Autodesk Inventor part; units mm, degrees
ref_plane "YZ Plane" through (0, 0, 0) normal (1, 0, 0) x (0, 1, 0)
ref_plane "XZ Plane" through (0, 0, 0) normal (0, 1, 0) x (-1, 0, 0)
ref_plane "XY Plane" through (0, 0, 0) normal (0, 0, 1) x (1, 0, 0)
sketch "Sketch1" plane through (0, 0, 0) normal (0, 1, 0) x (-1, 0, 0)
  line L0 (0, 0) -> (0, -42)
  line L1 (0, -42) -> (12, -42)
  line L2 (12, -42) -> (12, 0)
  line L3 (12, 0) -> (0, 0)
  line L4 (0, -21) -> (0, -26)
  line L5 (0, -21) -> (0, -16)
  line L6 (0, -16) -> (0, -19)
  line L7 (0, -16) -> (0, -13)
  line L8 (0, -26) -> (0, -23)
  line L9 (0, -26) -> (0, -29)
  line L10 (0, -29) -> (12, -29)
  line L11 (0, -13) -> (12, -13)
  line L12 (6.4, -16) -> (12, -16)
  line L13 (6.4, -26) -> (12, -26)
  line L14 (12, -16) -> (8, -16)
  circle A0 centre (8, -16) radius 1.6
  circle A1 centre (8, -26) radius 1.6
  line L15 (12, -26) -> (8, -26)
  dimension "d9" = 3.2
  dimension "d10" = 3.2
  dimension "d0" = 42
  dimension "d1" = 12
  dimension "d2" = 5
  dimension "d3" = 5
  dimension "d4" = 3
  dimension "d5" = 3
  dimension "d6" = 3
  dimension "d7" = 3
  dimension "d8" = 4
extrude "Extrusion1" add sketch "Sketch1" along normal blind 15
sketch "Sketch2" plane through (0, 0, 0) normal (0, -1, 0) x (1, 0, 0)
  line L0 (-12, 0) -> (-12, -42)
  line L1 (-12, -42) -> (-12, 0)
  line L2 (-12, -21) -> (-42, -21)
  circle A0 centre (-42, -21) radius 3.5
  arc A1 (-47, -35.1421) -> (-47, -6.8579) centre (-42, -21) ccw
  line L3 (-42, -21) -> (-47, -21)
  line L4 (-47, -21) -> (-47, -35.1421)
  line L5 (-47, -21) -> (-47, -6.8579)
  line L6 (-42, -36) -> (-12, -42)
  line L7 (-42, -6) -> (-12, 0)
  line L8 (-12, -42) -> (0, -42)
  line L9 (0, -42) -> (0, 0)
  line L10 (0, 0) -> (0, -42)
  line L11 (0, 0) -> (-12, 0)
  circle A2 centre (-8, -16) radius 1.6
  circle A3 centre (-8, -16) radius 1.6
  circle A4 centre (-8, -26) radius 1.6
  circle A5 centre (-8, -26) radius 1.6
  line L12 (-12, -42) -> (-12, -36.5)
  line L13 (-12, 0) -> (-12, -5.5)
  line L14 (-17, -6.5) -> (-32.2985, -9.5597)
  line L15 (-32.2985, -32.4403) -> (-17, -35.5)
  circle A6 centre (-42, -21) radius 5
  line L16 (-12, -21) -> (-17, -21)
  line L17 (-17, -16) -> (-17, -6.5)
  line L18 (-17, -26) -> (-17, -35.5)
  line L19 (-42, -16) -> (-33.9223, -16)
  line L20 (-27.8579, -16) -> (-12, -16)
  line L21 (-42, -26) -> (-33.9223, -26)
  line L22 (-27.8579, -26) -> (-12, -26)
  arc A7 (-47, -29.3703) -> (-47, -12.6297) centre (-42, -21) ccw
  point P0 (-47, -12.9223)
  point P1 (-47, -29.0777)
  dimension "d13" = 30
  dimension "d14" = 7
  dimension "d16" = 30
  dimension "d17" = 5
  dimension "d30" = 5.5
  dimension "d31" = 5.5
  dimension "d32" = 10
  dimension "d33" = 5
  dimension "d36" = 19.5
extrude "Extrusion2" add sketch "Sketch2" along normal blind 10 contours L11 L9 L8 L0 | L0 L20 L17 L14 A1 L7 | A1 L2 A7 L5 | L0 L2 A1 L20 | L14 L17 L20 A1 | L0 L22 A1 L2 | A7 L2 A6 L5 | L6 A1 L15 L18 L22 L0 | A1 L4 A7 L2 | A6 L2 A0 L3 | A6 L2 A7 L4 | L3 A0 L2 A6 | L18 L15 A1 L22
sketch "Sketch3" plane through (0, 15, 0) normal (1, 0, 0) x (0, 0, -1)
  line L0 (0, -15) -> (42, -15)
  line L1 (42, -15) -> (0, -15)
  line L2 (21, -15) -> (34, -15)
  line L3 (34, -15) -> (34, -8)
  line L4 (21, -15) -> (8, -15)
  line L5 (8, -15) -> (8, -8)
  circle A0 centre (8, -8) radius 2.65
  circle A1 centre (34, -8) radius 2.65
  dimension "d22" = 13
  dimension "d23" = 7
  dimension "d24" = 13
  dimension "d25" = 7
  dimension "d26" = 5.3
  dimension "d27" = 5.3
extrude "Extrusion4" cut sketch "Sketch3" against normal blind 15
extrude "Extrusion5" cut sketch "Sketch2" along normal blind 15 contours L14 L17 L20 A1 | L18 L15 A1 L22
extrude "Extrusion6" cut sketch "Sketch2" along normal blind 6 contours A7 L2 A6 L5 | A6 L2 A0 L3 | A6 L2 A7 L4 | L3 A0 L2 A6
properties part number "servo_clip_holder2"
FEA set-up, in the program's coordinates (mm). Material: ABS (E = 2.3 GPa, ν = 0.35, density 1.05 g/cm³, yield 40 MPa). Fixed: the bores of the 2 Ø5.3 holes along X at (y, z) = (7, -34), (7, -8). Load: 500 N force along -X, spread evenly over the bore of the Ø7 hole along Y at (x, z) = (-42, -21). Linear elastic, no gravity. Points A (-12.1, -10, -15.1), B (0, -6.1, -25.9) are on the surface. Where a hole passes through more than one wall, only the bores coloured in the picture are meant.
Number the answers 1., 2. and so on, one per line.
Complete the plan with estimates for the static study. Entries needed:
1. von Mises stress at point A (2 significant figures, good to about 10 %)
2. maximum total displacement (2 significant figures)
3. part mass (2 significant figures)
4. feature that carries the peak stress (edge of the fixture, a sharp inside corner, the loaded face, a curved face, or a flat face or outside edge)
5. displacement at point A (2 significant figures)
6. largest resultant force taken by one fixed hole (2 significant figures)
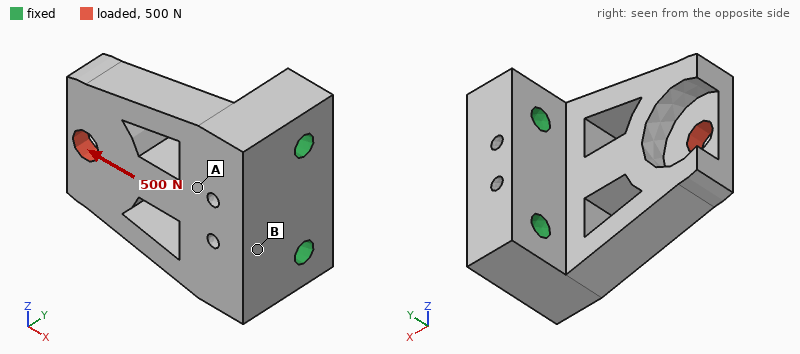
1. 4.8 MPa
2. 0.50 mm
3. 21 g
4. a flat face or outside edge
5. 0.092 mm
6. 250 N
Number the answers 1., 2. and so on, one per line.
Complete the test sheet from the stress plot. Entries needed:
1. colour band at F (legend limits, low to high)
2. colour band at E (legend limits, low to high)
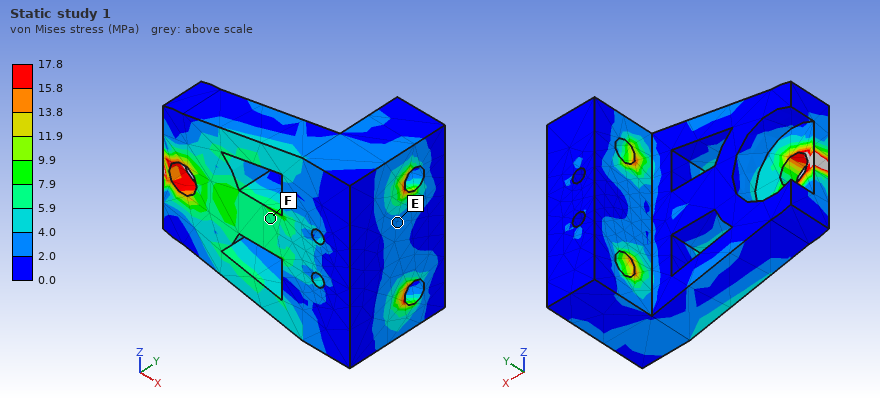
1. 5.9 to 7.9 MPa
2. 2.0 to 4.0 MPa
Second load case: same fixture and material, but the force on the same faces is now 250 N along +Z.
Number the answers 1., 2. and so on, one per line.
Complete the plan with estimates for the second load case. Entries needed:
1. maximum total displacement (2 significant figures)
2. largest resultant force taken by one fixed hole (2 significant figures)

1. 0.22 mm
2. 320 N
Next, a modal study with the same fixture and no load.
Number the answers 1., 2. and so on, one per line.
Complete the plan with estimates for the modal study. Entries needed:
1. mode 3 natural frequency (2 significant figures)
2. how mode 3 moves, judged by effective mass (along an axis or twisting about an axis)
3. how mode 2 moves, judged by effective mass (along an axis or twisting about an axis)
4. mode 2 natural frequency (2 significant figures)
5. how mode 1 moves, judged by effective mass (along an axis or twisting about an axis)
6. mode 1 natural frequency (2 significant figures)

1. 3000 Hz
2. along Z
3. along Z
4. 2700 Hz
5. along Y
6. 1400 Hz
